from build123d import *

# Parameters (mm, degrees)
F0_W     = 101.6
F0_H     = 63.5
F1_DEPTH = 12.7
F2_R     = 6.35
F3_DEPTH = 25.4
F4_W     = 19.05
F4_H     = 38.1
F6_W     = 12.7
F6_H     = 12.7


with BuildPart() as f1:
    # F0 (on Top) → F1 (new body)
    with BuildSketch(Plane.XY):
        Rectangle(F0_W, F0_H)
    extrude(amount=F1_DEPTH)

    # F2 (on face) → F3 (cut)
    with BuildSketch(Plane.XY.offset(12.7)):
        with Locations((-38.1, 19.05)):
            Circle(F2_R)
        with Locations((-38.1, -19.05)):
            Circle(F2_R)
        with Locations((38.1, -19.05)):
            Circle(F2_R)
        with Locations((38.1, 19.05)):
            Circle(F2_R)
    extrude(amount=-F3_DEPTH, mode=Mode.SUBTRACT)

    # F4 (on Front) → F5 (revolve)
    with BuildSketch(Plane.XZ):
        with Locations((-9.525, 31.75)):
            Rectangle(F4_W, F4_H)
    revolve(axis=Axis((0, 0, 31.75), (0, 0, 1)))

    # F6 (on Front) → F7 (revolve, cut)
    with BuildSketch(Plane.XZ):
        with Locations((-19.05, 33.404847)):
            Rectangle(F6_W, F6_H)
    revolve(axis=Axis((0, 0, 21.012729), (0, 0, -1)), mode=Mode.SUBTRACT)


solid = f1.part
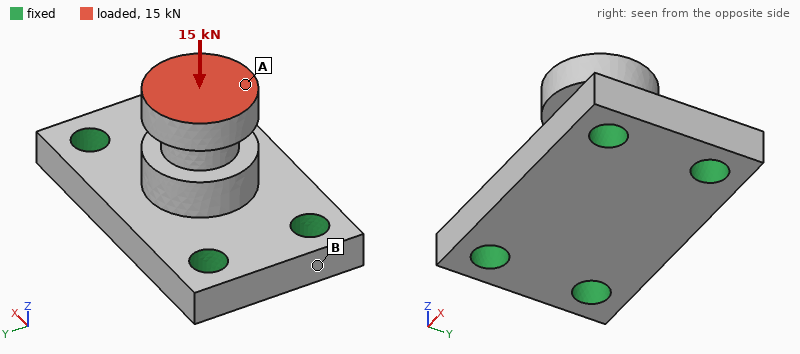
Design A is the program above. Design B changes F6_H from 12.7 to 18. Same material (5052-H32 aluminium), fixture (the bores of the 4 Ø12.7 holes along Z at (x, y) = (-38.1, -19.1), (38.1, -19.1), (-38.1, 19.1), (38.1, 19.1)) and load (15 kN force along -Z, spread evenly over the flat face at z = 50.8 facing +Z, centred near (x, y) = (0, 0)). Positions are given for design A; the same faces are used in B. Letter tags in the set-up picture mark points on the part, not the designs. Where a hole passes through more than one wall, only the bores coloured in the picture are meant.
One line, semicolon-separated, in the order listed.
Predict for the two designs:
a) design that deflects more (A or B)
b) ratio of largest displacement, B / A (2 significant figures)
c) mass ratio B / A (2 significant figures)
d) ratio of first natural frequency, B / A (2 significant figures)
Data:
B; 1.1; 0.97; 1.0
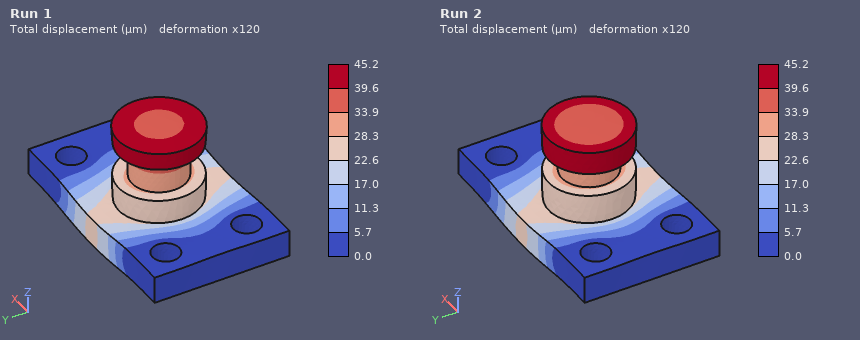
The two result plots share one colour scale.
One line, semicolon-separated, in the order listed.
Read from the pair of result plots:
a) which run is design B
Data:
Run 1
